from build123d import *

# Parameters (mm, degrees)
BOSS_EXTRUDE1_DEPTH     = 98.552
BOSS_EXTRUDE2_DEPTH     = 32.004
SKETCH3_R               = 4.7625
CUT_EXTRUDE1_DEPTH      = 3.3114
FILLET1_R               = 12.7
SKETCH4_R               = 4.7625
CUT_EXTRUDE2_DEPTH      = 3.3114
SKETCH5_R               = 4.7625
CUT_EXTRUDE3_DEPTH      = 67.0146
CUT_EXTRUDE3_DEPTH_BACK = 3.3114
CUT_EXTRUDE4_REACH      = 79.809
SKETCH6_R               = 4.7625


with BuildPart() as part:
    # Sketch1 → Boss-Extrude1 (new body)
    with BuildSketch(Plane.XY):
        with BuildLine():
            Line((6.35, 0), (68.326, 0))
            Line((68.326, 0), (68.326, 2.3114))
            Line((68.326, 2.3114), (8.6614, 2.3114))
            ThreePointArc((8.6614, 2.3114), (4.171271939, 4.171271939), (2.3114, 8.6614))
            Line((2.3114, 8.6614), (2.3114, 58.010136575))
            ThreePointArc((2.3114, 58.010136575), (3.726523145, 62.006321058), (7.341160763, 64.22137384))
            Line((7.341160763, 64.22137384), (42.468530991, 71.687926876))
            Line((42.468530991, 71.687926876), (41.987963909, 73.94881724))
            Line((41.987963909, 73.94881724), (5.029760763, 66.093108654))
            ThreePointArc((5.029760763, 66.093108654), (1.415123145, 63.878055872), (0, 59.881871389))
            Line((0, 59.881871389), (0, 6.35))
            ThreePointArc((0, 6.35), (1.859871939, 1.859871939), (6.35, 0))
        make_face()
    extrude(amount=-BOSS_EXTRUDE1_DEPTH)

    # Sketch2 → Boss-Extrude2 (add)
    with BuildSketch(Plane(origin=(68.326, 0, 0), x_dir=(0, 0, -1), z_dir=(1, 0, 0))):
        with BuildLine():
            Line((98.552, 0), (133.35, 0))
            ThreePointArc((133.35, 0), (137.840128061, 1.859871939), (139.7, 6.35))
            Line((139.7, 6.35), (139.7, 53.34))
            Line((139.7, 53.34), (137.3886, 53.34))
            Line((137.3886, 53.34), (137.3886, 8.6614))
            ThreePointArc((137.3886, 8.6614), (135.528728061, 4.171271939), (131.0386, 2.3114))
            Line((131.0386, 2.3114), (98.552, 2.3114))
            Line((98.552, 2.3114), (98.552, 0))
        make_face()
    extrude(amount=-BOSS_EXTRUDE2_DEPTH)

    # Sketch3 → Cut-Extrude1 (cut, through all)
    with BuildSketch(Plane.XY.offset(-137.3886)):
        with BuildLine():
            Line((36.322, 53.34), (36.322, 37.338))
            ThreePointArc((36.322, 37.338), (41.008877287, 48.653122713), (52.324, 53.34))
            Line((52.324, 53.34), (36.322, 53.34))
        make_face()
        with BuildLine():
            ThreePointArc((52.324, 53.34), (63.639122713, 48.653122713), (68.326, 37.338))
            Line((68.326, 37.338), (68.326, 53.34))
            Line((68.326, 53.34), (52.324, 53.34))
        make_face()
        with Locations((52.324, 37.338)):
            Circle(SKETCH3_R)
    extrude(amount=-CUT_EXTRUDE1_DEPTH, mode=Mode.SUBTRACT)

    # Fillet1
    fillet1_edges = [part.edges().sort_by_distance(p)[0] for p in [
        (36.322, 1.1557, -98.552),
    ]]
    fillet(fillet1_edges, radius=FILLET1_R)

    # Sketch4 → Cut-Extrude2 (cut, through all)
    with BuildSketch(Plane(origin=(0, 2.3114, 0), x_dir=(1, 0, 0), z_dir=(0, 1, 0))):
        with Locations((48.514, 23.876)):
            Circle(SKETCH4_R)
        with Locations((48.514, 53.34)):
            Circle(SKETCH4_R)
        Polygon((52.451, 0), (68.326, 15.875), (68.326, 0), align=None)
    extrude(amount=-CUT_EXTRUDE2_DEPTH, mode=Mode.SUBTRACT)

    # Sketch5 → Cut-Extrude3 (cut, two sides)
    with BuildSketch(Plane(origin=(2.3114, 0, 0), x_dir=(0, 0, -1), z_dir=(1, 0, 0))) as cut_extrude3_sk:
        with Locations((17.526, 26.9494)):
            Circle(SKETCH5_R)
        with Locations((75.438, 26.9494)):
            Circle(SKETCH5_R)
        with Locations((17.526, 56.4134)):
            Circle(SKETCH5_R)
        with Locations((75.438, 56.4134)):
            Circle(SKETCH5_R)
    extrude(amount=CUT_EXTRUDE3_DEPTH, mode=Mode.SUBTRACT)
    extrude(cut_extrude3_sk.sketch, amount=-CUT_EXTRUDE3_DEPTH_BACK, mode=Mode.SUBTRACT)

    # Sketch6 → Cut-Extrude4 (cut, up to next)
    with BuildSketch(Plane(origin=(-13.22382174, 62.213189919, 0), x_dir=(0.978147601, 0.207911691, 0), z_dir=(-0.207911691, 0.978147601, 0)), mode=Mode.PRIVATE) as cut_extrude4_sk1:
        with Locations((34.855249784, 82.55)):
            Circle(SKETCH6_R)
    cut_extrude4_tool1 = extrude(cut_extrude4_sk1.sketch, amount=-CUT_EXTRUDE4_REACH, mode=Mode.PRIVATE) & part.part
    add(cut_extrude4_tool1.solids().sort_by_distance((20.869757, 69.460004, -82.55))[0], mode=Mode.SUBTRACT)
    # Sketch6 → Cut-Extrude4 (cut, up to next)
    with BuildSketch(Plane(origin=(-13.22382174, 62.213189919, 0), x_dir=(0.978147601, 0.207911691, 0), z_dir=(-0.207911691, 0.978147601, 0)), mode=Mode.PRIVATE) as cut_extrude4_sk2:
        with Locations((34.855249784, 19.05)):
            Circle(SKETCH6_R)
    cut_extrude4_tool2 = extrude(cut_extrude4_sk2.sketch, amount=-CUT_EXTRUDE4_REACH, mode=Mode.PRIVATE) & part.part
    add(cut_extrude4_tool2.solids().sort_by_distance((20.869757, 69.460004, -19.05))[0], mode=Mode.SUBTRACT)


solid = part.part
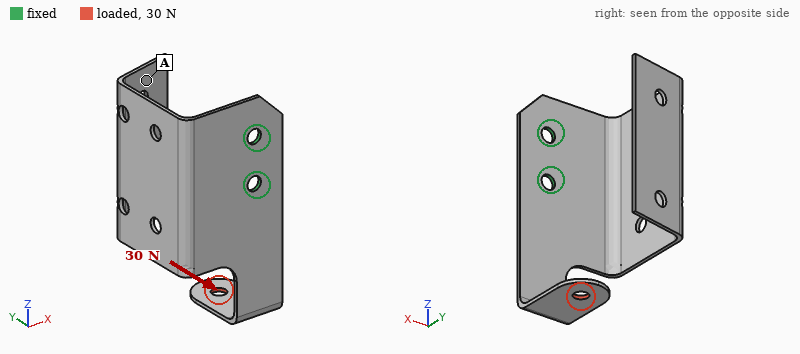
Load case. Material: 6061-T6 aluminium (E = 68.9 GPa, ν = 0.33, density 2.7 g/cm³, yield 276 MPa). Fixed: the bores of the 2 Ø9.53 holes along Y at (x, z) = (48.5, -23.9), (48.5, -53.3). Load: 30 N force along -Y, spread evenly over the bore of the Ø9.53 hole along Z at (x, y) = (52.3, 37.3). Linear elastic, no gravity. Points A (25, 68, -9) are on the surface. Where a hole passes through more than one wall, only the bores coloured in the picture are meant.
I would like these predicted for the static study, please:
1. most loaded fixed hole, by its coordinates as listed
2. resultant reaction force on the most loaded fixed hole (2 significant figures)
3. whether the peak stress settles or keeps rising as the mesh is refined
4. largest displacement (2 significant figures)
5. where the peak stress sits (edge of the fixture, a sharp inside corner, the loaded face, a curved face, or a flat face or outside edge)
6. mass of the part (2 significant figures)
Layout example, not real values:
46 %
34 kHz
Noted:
(48.5, -53.3)
60 N
keeps rising
2.0 mm
edge of the fixture
120 g
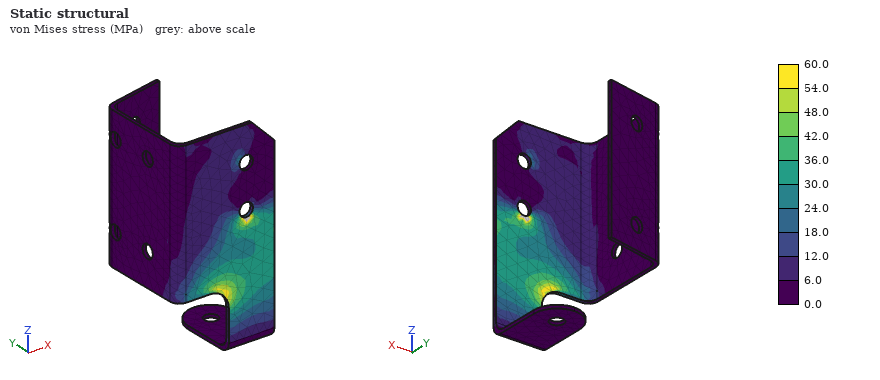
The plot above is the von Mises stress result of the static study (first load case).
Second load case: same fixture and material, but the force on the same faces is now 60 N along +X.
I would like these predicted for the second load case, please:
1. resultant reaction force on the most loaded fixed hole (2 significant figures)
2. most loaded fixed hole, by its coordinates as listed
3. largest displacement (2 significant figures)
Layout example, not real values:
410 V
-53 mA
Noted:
180 N
(48.5, -53.3)
2.0 mm
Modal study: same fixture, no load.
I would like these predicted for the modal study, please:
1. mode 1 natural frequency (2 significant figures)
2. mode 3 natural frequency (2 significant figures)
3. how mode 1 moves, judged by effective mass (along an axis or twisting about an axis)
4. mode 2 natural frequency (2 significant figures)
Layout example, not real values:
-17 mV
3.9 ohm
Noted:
130 Hz
220 Hz
along X
180 Hz
